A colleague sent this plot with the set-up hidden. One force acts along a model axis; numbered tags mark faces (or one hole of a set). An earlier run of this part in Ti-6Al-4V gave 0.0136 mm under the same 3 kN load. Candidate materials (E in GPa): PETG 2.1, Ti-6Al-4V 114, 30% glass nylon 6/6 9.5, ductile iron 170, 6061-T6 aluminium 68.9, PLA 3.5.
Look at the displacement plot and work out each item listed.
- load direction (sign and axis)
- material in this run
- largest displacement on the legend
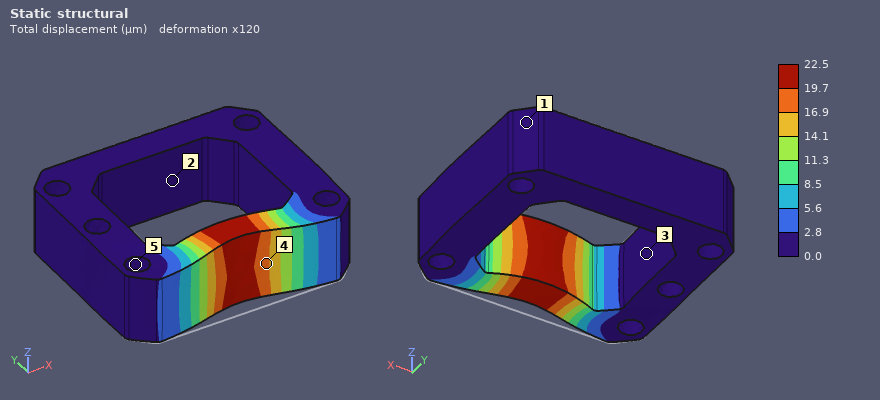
+Y
6061-T6 aluminium
22.5 µm
